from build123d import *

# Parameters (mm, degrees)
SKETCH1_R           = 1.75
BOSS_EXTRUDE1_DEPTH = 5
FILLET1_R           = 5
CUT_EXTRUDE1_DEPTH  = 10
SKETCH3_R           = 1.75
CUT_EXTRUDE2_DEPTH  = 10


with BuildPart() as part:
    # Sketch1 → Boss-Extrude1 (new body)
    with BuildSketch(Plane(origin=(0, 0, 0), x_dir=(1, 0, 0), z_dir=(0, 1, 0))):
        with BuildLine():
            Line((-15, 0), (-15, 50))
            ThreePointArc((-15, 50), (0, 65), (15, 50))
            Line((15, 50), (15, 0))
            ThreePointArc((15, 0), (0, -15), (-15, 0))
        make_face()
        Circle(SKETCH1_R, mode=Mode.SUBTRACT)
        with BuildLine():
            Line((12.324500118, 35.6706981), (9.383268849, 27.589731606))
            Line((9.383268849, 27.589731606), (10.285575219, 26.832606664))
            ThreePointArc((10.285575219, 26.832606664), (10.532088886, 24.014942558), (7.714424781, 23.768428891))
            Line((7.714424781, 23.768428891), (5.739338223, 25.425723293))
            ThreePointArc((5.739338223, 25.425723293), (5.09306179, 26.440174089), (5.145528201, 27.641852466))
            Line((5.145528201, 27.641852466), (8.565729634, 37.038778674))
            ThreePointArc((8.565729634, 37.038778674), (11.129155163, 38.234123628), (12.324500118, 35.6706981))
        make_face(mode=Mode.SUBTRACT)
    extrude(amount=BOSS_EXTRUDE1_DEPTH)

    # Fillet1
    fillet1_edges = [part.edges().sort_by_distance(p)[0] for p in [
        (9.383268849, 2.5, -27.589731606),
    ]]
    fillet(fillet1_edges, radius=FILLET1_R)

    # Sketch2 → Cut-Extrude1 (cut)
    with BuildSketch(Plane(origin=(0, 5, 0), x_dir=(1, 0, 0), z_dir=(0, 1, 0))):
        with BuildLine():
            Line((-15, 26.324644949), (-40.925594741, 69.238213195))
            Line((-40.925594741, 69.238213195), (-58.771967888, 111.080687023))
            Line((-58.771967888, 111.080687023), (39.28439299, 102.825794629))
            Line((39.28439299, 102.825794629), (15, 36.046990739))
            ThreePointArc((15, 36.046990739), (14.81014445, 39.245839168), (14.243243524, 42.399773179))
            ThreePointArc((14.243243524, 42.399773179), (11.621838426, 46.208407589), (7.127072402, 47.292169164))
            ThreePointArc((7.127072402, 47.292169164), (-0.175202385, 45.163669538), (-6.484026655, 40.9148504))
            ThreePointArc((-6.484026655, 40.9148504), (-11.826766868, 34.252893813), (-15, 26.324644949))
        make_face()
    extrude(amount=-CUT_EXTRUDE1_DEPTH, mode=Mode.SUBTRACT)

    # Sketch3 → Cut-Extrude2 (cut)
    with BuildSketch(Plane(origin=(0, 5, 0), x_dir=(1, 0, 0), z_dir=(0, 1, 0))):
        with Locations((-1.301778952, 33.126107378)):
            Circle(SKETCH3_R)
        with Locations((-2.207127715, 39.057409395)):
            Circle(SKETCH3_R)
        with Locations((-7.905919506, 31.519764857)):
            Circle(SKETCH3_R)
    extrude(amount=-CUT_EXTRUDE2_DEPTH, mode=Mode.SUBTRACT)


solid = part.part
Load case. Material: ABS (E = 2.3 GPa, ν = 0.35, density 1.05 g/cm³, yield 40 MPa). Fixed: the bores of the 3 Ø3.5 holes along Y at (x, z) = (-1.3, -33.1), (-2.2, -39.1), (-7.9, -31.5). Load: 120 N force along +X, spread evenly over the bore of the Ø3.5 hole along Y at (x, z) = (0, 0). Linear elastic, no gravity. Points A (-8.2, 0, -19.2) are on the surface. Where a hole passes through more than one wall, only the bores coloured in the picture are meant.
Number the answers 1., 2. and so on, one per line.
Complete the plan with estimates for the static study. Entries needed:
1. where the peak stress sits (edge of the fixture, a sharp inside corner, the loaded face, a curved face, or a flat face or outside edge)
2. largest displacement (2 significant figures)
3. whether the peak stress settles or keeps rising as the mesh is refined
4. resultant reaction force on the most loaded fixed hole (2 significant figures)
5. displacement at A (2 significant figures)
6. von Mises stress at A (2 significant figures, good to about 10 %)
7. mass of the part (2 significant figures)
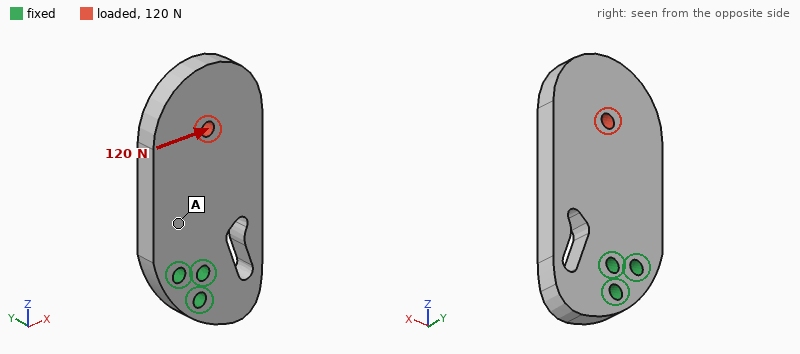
1. edge of the fixture
2. 0.32 mm
3. keeps rising
4. 310 N
5. 0.075 mm
6. 3.1 MPa
7. 8.0 g
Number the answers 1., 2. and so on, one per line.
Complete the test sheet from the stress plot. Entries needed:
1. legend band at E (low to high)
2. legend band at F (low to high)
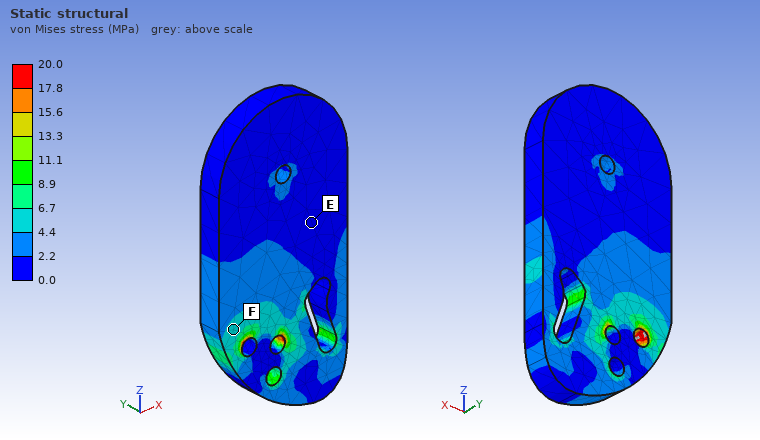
1. 0.0 to 2.2 MPa
2. 4.4 to 6.7 MPa
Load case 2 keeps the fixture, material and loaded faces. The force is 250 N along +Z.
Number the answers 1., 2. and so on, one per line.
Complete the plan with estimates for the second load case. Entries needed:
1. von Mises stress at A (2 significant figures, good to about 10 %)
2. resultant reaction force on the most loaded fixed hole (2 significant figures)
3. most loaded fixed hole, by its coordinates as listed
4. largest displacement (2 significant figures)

1. 1.8 MPa
2. 190 N
3. (-1.3, -33.1)
4. 91 µm
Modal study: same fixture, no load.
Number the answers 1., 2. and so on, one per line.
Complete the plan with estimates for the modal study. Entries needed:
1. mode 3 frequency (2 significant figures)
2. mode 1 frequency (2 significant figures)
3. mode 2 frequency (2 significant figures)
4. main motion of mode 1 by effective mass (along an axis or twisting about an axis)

1. 1700 Hz
2. 560 Hz
3. 1700 Hz
4. along Y
